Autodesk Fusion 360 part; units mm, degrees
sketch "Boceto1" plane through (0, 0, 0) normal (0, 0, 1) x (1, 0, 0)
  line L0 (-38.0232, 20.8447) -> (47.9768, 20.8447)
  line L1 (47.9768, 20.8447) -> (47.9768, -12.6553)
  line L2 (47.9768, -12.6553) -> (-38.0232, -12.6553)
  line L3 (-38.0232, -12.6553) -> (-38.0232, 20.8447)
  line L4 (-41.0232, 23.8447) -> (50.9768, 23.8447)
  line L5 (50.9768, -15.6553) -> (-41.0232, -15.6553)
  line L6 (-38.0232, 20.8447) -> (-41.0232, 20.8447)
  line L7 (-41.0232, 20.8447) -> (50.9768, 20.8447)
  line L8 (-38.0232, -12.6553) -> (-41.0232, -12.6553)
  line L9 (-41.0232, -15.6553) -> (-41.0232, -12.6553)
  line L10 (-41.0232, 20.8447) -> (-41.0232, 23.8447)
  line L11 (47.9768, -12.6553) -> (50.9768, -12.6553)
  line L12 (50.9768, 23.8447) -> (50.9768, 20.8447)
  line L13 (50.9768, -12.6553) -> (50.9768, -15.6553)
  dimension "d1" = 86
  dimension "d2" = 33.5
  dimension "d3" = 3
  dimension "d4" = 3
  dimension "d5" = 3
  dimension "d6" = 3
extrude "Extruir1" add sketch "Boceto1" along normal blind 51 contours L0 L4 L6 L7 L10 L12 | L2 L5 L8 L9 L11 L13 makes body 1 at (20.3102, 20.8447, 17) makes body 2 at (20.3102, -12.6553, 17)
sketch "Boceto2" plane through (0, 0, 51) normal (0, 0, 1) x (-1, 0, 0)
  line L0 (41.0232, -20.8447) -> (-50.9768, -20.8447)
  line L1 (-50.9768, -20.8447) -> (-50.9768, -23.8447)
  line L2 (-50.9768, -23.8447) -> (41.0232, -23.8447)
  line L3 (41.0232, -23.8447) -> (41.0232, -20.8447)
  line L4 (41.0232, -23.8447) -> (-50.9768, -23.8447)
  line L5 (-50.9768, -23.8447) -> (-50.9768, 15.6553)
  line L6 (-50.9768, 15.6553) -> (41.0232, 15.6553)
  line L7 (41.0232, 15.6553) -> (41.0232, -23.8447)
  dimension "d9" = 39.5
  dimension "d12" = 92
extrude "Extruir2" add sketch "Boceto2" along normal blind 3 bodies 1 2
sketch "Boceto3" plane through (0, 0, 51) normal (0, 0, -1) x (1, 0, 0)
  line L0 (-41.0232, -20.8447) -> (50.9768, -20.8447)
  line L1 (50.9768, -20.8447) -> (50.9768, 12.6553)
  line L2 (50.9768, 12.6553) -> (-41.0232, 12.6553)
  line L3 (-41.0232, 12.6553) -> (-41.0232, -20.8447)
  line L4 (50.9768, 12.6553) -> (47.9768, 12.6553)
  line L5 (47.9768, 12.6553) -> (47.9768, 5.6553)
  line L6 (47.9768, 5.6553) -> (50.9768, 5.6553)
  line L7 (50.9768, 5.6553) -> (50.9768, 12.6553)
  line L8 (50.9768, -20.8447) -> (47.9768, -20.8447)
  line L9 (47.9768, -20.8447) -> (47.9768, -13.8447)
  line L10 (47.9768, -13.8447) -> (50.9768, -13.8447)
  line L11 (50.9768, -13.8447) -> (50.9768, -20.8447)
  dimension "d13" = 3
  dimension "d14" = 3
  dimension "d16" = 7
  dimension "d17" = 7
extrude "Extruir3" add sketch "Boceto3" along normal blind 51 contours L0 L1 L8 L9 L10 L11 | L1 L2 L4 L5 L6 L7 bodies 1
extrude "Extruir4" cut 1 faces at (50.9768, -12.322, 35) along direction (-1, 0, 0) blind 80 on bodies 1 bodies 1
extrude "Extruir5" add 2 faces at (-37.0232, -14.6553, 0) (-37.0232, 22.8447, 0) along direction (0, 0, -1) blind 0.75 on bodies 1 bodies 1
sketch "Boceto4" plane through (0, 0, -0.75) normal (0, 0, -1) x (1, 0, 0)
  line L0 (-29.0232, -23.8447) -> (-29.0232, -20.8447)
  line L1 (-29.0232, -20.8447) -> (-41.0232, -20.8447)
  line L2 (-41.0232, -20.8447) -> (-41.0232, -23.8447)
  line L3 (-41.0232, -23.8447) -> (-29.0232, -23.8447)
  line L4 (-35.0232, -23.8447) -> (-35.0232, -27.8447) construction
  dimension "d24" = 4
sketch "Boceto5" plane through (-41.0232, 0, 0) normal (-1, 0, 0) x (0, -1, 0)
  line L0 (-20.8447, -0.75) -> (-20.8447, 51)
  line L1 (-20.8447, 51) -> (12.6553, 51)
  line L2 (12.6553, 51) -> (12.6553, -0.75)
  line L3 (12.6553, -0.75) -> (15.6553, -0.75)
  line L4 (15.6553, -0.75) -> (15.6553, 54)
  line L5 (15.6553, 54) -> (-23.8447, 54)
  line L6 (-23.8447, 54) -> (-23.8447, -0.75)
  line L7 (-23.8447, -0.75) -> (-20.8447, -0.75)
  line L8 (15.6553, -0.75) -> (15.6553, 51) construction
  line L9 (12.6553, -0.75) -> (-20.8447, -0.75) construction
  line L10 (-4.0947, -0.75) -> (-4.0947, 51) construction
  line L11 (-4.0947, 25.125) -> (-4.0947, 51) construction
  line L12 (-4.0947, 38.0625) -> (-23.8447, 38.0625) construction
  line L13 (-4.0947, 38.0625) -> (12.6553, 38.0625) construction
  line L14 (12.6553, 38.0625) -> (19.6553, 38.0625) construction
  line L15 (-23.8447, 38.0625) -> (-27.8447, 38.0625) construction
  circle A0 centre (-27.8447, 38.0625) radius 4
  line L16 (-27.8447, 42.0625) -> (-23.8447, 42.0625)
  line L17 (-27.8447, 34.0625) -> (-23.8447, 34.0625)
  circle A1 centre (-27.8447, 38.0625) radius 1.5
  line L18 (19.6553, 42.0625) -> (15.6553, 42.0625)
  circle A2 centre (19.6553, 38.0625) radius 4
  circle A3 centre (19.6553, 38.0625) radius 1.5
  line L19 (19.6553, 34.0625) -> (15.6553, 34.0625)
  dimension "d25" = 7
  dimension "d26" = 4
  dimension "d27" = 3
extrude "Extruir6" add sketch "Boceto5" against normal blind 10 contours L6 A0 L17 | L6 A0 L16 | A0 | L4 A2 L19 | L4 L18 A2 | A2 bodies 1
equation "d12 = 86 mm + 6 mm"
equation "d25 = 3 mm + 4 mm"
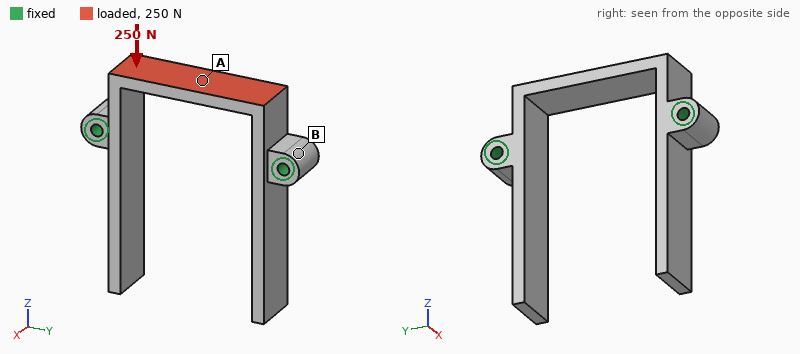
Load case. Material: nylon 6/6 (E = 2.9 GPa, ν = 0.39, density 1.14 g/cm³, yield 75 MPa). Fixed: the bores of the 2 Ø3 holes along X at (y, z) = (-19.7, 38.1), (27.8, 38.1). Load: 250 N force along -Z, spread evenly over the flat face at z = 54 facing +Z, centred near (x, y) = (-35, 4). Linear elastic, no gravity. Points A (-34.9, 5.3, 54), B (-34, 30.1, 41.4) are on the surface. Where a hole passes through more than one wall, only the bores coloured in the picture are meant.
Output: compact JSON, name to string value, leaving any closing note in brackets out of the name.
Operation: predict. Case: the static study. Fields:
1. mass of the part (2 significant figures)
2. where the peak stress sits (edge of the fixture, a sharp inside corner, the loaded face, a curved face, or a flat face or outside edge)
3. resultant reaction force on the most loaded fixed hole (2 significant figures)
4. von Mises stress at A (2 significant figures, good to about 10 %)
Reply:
{"mass of the part": "7.0 g", "where the peak stress sits": "a flat face or outside edge", "resultant reaction force on the most loaded fixed hole": "150 N", "von Mises stress at A": "23 MPa"}
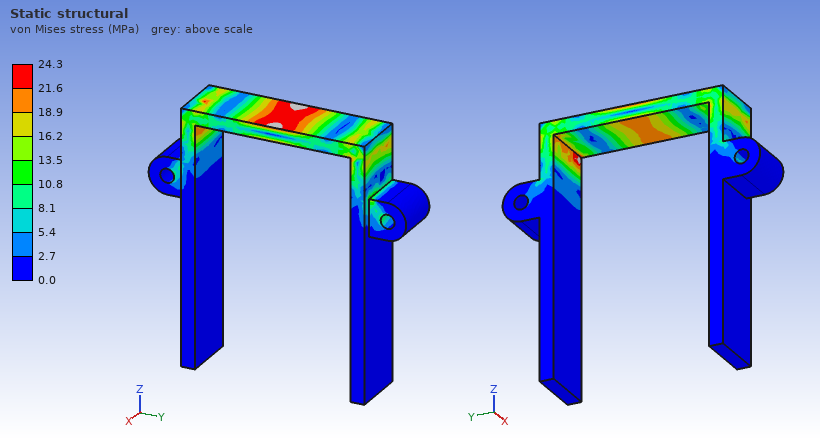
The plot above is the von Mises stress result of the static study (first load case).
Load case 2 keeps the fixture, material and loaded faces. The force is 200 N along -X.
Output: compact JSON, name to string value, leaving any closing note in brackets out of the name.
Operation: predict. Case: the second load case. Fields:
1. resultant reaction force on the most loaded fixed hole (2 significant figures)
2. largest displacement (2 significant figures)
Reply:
{"resultant reaction force on the most loaded fixed hole": "100 N", "largest displacement": "0.37 mm"}
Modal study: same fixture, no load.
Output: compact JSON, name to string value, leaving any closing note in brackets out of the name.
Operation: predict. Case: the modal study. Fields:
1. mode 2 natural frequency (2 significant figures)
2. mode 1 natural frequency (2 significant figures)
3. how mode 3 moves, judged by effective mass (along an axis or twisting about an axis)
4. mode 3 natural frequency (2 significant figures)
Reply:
{"mode 2 natural frequency": "570 Hz", "mode 1 natural frequency": "570 Hz", "how mode 3 moves, judged by effective mass": "along X", "mode 3 natural frequency": "1600 Hz"}
